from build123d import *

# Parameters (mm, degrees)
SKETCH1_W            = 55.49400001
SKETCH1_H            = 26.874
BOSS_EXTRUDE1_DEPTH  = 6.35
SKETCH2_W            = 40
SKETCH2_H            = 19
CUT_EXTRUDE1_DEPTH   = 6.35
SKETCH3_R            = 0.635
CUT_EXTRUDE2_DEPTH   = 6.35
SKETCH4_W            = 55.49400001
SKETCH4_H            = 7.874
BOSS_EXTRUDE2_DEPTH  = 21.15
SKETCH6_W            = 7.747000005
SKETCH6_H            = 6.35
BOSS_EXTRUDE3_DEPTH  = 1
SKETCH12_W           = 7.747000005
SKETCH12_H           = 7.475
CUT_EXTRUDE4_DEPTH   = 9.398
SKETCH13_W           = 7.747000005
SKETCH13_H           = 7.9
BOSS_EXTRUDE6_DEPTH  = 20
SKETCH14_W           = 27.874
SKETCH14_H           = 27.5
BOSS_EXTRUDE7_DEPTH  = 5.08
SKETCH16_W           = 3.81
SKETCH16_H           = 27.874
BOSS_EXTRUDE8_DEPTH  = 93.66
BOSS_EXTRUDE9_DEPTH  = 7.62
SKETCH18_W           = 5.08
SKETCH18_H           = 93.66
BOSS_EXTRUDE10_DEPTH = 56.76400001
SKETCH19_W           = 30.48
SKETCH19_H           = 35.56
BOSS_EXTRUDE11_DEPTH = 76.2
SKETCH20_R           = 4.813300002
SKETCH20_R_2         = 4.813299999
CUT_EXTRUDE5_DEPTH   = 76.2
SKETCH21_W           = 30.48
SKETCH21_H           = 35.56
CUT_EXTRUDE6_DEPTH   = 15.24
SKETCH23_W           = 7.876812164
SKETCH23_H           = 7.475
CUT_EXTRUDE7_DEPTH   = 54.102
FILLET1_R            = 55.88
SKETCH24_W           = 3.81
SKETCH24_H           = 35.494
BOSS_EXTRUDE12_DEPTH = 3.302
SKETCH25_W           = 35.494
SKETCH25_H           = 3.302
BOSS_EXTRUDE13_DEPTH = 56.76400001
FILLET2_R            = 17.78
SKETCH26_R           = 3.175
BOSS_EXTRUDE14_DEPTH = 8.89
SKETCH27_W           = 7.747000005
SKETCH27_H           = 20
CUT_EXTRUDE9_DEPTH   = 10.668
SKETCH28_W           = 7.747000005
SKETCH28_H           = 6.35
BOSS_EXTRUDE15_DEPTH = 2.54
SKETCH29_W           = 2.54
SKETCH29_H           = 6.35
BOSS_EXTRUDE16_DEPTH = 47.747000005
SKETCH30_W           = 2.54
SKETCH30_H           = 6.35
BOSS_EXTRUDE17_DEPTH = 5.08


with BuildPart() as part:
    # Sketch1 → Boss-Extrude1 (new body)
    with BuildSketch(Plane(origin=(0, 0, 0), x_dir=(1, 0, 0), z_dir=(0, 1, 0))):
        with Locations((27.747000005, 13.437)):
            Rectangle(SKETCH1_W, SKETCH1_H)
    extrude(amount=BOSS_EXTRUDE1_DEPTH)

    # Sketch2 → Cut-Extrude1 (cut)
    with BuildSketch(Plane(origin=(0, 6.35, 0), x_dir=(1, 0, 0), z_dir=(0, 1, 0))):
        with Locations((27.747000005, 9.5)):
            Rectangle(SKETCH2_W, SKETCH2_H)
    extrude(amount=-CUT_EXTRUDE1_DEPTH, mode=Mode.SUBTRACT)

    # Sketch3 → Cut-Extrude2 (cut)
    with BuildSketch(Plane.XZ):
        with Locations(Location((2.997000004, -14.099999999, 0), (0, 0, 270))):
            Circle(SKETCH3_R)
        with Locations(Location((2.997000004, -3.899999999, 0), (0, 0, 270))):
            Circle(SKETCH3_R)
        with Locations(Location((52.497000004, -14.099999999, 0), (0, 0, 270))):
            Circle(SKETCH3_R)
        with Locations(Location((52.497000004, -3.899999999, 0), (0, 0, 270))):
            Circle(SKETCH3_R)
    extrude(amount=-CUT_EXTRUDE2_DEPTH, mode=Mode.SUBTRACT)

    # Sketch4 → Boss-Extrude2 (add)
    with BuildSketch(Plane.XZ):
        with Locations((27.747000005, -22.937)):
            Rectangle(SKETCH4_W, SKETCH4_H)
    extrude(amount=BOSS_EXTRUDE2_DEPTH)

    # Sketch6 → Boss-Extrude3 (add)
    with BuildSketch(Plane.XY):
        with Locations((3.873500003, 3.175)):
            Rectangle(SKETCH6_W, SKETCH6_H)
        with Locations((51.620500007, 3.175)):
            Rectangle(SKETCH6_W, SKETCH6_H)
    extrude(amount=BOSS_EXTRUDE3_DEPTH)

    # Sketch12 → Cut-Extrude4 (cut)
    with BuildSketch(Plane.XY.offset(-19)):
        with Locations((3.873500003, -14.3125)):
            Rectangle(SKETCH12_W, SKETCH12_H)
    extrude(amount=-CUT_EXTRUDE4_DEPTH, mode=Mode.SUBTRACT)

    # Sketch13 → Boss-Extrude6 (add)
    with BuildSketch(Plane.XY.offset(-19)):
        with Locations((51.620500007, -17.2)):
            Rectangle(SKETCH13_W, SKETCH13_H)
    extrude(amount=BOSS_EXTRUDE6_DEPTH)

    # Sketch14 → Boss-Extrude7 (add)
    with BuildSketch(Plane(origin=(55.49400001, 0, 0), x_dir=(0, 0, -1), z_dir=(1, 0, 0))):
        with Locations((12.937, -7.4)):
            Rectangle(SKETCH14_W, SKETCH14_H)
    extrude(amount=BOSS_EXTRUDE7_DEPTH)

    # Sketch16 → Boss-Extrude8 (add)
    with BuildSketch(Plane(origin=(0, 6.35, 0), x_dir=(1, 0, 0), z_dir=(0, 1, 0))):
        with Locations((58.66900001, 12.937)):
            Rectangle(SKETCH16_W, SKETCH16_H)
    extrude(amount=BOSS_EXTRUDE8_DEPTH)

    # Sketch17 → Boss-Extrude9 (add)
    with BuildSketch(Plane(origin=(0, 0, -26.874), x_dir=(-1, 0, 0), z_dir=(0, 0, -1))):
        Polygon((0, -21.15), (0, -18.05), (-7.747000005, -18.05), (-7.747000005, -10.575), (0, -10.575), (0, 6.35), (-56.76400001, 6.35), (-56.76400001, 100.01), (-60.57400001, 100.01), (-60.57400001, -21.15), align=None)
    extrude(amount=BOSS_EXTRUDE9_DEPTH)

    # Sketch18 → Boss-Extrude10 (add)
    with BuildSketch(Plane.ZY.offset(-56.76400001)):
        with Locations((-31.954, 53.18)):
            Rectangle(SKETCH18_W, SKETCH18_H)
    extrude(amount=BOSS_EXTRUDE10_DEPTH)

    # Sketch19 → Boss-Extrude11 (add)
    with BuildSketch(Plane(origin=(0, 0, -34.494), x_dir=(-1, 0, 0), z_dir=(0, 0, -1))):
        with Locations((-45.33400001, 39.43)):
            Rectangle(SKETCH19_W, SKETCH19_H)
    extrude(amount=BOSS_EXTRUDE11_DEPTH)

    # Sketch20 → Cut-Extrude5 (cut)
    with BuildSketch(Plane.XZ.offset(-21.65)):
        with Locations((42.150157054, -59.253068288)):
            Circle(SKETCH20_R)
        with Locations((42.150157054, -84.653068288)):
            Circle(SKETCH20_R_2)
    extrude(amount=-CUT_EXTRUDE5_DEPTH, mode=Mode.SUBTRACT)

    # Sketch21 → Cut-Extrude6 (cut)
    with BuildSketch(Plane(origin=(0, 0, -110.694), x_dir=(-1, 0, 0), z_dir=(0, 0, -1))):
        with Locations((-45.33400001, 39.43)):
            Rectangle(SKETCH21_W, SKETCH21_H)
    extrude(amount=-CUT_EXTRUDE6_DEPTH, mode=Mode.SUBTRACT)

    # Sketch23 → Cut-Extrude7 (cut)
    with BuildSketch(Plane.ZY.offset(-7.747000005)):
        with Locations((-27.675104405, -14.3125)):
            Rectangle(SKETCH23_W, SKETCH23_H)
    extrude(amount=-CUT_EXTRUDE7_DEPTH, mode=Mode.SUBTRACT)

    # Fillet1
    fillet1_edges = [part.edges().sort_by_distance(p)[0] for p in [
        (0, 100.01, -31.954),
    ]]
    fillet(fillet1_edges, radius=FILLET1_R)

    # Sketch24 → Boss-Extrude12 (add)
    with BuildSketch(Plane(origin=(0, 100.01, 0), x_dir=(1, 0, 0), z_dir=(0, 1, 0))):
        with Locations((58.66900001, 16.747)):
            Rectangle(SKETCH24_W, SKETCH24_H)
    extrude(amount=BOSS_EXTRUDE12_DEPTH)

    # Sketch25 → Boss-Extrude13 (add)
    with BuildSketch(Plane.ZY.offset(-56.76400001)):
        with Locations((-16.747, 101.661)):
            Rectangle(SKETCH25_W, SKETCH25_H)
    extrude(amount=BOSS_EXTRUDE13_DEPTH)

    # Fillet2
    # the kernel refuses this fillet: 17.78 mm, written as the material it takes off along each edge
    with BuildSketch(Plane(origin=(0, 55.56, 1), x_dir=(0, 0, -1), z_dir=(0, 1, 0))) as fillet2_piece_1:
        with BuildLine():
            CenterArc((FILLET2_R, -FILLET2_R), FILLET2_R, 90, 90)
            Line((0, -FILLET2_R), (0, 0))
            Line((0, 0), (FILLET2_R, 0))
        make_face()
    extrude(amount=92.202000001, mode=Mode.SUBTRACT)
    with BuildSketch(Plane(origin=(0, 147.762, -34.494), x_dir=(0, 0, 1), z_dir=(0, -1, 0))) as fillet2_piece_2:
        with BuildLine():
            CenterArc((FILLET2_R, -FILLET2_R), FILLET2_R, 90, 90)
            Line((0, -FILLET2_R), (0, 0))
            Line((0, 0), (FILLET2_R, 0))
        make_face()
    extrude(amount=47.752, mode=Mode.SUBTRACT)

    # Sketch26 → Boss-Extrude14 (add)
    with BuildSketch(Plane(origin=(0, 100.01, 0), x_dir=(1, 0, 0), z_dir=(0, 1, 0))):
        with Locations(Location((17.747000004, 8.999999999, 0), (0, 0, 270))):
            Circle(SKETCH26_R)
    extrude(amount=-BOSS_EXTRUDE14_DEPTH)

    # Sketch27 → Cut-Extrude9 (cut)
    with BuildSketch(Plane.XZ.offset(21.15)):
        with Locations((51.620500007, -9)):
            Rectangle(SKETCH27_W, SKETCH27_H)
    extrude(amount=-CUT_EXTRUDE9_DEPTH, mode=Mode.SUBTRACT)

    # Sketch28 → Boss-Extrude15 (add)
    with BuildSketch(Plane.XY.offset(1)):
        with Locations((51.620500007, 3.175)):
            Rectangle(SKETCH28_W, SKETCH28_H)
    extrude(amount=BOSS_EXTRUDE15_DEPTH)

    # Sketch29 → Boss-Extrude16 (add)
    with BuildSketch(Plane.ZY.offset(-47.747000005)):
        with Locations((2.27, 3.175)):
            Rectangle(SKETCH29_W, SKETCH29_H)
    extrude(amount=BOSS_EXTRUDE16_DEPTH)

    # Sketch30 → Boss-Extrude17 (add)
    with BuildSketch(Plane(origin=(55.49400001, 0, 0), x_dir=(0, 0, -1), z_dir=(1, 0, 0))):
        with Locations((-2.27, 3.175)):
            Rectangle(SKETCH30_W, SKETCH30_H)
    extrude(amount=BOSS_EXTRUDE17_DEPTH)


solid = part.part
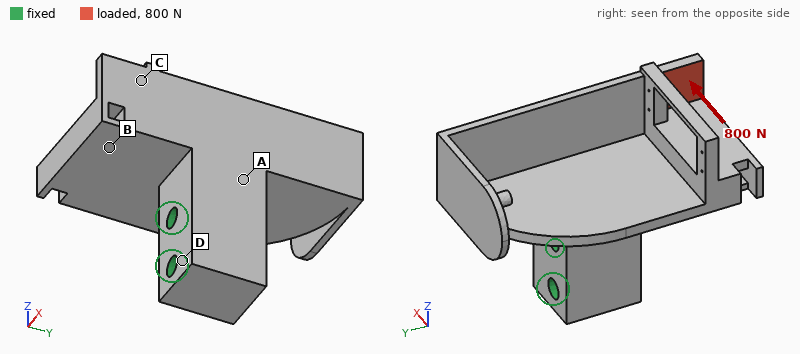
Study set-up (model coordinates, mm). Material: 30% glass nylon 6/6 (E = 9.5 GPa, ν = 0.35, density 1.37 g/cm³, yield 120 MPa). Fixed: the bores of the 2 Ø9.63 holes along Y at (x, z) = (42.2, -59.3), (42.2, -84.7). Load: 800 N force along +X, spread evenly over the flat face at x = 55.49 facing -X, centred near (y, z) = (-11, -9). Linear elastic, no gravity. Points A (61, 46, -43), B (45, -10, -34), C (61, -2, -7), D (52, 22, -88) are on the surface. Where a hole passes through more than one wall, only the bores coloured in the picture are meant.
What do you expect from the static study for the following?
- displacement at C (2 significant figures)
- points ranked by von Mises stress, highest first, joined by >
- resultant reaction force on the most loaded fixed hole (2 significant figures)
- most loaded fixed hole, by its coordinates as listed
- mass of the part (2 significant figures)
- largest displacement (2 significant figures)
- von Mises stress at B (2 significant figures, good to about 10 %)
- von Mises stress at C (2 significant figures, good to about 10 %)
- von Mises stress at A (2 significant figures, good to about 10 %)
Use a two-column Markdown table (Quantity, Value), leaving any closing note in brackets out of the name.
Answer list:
| Quantity | Value |
|---|---|
| displacement at C | 0.53 mm |
| points ranked by von Mises stress, highest first, joined by > | C > A > B > D |
| resultant reaction force on the most loaded fixed hole | 1.6 kN |
| most loaded fixed hole, by its coordinates as listed | (42.2, -59.3) |
| mass of the part | 180 g |
| largest displacement | 0.96 mm |
| von Mises stress at B | 6.5 MPa |
| von Mises stress at C | 20 MPa |
| von Mises stress at A | 9.0 MPa |
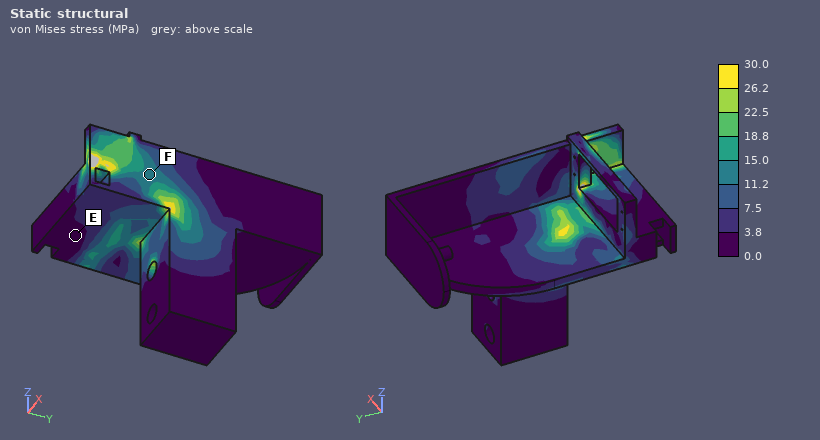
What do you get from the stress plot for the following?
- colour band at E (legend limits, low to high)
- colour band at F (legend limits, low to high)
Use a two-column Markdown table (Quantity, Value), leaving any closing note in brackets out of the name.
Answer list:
| Quantity | Value |
|---|---|
| colour band at E | 0.0 to 3.8 MPa |
| colour band at F | 11.2 to 15.0 MPa |
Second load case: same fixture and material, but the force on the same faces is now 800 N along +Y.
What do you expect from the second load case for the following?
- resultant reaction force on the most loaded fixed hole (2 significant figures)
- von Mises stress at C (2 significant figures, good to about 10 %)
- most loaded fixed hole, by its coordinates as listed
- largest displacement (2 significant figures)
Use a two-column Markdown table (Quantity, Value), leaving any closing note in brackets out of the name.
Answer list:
| Quantity | Value |
|---|---|
| resultant reaction force on the most loaded fixed hole | 940 N |
| von Mises stress at C | 5.9 MPa |
| most loaded fixed hole, by its coordinates as listed | (42.2, -59.3) |
| largest displacement | 0.30 mm |
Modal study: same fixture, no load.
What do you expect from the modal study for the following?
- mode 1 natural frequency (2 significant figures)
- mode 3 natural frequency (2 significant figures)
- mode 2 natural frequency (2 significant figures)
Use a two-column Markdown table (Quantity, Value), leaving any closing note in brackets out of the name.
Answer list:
| Quantity | Value |
|---|---|
| mode 1 natural frequency | 370 Hz |
| mode 3 natural frequency | 970 Hz |
| mode 2 natural frequency | 500 Hz |
